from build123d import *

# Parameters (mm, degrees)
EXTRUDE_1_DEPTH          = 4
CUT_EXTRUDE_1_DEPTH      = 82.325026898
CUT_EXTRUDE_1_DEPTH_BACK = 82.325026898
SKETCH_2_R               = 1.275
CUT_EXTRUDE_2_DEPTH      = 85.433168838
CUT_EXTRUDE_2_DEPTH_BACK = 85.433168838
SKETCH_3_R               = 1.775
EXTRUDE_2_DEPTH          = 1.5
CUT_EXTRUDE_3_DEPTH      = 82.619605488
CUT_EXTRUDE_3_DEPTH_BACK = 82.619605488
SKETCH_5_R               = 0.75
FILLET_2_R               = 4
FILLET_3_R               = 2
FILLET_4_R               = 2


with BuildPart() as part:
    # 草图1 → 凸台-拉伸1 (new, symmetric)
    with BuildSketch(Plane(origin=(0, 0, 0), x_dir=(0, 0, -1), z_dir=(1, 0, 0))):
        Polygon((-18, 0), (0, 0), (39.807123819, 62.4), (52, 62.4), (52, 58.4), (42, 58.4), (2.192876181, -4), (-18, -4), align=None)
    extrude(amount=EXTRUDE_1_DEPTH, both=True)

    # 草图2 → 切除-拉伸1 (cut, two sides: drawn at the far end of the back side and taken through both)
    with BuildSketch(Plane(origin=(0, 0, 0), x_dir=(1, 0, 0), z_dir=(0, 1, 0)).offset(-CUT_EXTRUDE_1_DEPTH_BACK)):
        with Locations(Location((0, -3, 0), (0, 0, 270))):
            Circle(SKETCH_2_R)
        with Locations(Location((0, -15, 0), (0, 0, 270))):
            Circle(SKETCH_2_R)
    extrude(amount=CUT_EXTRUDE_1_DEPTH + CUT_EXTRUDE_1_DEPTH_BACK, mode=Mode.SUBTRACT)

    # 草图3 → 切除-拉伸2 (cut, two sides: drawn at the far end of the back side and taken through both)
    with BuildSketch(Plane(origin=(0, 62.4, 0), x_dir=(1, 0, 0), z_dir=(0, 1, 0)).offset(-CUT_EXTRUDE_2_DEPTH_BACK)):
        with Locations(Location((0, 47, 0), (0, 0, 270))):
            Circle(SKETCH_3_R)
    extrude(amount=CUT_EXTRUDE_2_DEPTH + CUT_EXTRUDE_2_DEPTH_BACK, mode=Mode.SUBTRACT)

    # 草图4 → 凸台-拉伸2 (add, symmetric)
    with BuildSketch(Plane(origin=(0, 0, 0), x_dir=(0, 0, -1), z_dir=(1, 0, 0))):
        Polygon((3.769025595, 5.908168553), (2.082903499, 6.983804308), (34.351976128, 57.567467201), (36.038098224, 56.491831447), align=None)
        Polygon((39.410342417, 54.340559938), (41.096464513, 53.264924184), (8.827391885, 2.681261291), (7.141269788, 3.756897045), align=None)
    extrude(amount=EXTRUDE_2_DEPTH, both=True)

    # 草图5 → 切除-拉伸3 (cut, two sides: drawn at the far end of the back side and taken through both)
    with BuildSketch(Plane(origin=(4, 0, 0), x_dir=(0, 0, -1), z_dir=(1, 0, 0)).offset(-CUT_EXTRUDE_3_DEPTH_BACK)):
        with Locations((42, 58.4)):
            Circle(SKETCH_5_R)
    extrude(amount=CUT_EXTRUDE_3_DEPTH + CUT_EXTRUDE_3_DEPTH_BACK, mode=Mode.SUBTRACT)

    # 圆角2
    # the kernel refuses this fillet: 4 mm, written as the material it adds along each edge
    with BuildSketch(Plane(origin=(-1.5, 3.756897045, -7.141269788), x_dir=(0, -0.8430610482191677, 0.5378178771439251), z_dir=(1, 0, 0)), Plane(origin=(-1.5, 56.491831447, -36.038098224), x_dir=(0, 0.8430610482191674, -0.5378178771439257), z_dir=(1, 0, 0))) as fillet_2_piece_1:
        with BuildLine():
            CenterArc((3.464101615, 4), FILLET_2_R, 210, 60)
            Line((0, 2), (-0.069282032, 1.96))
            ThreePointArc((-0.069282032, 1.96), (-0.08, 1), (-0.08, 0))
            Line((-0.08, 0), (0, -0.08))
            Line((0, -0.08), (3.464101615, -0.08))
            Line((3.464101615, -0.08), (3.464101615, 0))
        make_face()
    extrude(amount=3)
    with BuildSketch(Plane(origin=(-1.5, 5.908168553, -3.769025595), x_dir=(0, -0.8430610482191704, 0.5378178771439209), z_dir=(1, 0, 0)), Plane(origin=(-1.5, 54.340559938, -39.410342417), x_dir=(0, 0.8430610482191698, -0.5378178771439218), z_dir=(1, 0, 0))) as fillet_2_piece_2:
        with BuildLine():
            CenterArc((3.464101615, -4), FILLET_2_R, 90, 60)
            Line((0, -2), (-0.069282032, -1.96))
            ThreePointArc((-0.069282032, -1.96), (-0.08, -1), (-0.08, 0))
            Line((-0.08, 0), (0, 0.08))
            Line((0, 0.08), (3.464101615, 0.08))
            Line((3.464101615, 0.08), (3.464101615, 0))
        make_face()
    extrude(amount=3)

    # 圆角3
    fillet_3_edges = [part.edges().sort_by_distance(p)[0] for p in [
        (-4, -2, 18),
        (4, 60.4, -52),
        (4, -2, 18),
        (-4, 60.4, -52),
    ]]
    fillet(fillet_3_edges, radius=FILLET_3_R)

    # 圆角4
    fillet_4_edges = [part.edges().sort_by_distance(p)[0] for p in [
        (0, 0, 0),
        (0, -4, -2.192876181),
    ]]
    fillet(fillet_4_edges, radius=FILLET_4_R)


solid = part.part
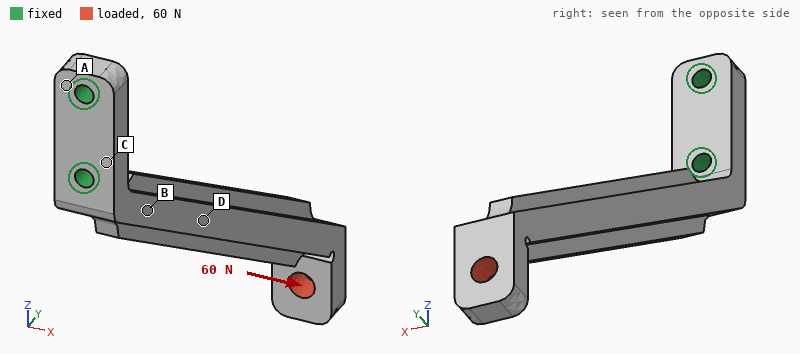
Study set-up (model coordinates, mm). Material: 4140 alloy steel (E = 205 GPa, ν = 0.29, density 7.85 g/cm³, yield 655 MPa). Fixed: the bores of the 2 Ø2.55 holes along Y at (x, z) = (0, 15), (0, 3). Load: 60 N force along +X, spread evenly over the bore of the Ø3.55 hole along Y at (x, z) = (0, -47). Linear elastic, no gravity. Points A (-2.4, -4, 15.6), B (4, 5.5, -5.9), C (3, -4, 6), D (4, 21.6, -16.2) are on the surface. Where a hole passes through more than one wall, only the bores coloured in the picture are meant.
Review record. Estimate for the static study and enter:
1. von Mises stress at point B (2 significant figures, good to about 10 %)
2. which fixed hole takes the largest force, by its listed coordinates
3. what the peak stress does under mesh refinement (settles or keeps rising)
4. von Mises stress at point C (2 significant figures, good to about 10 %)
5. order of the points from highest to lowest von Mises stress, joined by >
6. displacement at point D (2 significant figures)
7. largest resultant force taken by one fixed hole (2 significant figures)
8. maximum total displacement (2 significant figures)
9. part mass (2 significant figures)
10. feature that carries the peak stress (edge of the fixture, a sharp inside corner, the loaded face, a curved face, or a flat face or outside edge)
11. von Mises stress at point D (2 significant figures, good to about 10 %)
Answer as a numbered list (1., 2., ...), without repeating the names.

1. 94 MPa
2. (0, 3)
3. keeps rising
4. 35 MPa
5. B > D > C > A
6. 0.081 mm
7. 180 N
8. 0.38 mm
9. 31 g
10. edge of the fixture
11. 66 MPa
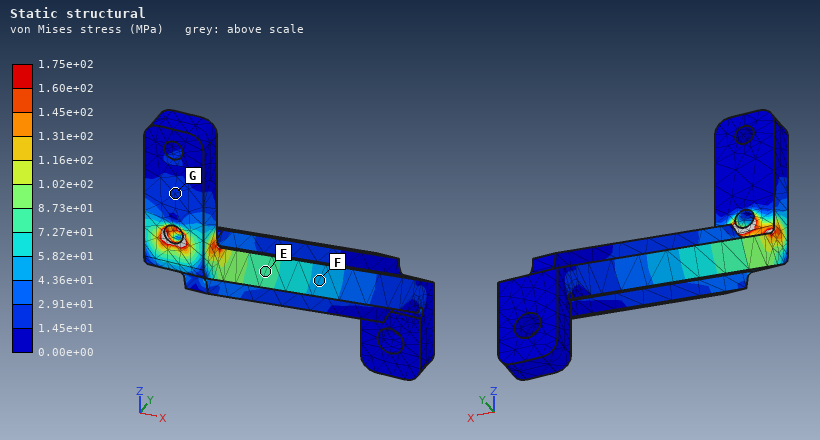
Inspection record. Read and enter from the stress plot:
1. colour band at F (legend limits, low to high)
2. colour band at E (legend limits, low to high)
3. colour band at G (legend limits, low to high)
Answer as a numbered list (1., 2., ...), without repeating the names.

1. 4.36e+01 to 5.82e+01 MPa
2. 7.27e+01 to 8.73e+01 MPa
3. 1.45e+01 to 2.91e+01 MPa
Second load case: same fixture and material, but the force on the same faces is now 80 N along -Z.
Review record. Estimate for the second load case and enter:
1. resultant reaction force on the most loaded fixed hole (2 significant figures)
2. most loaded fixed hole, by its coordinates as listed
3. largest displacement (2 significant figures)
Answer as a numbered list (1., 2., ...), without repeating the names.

1. 100 N
2. (0, 3)
3. 0.71 mm
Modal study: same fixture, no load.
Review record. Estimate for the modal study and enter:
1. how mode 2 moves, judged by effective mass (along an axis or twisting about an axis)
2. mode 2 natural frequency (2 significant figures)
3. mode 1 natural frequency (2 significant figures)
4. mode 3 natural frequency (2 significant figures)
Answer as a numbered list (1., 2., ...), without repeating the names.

1. along X
2. 740 Hz
3. 540 Hz
4. 4000 Hz
